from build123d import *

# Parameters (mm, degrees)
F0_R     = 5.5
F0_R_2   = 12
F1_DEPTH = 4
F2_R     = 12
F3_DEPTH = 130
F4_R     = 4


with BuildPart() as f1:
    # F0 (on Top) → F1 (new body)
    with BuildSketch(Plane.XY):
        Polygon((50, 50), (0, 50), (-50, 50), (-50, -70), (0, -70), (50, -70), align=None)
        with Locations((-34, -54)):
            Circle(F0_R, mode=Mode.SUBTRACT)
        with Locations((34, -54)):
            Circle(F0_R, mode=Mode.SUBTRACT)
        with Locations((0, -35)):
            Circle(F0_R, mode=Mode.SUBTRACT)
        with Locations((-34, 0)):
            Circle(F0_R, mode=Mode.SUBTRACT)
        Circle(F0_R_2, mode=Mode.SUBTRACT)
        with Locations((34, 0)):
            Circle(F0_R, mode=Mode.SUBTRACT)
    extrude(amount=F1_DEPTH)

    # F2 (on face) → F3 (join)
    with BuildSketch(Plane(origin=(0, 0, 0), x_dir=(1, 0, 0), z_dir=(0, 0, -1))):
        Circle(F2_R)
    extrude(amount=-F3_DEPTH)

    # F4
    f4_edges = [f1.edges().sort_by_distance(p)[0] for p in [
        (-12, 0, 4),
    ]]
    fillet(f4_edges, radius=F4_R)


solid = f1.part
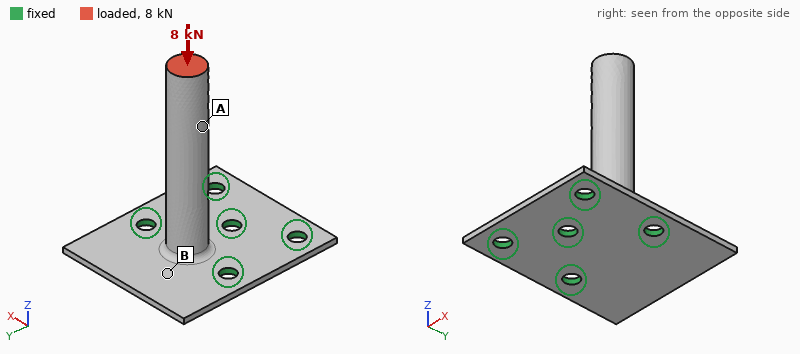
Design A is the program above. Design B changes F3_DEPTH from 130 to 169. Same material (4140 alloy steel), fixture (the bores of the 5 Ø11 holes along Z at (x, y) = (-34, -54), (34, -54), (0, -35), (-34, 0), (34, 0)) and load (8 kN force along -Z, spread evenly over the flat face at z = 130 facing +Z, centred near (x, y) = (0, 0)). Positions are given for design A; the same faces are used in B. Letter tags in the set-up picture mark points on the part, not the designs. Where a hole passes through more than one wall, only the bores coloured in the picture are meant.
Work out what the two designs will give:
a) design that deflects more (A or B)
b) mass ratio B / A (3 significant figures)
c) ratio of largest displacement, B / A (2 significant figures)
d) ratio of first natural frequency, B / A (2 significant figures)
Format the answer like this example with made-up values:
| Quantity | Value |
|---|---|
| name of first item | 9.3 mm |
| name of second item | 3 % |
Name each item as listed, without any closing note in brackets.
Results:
| Quantity | Value |
|---|---|
| design that deflects more | B |
| mass ratio B / A | 1.17 |
| ratio of largest displacement, B / A | 1.3 |
| ratio of first natural frequency, B / A | 0.66 |
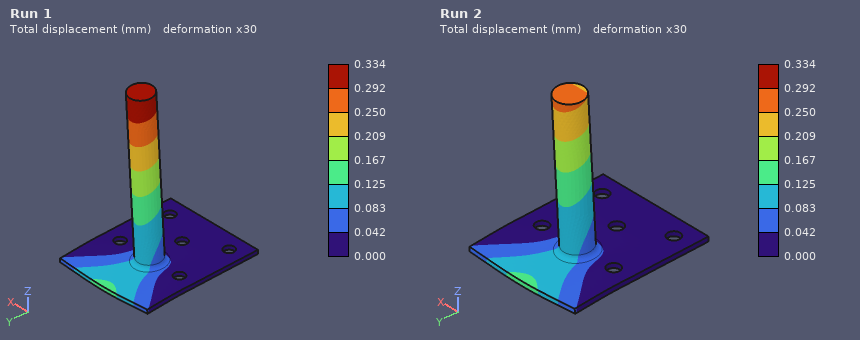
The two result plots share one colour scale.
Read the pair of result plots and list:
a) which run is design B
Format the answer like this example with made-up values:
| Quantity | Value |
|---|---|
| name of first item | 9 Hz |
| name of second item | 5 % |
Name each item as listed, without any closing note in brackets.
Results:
| Quantity | Value |
|---|---|
| which run is design B | Run 1 |
